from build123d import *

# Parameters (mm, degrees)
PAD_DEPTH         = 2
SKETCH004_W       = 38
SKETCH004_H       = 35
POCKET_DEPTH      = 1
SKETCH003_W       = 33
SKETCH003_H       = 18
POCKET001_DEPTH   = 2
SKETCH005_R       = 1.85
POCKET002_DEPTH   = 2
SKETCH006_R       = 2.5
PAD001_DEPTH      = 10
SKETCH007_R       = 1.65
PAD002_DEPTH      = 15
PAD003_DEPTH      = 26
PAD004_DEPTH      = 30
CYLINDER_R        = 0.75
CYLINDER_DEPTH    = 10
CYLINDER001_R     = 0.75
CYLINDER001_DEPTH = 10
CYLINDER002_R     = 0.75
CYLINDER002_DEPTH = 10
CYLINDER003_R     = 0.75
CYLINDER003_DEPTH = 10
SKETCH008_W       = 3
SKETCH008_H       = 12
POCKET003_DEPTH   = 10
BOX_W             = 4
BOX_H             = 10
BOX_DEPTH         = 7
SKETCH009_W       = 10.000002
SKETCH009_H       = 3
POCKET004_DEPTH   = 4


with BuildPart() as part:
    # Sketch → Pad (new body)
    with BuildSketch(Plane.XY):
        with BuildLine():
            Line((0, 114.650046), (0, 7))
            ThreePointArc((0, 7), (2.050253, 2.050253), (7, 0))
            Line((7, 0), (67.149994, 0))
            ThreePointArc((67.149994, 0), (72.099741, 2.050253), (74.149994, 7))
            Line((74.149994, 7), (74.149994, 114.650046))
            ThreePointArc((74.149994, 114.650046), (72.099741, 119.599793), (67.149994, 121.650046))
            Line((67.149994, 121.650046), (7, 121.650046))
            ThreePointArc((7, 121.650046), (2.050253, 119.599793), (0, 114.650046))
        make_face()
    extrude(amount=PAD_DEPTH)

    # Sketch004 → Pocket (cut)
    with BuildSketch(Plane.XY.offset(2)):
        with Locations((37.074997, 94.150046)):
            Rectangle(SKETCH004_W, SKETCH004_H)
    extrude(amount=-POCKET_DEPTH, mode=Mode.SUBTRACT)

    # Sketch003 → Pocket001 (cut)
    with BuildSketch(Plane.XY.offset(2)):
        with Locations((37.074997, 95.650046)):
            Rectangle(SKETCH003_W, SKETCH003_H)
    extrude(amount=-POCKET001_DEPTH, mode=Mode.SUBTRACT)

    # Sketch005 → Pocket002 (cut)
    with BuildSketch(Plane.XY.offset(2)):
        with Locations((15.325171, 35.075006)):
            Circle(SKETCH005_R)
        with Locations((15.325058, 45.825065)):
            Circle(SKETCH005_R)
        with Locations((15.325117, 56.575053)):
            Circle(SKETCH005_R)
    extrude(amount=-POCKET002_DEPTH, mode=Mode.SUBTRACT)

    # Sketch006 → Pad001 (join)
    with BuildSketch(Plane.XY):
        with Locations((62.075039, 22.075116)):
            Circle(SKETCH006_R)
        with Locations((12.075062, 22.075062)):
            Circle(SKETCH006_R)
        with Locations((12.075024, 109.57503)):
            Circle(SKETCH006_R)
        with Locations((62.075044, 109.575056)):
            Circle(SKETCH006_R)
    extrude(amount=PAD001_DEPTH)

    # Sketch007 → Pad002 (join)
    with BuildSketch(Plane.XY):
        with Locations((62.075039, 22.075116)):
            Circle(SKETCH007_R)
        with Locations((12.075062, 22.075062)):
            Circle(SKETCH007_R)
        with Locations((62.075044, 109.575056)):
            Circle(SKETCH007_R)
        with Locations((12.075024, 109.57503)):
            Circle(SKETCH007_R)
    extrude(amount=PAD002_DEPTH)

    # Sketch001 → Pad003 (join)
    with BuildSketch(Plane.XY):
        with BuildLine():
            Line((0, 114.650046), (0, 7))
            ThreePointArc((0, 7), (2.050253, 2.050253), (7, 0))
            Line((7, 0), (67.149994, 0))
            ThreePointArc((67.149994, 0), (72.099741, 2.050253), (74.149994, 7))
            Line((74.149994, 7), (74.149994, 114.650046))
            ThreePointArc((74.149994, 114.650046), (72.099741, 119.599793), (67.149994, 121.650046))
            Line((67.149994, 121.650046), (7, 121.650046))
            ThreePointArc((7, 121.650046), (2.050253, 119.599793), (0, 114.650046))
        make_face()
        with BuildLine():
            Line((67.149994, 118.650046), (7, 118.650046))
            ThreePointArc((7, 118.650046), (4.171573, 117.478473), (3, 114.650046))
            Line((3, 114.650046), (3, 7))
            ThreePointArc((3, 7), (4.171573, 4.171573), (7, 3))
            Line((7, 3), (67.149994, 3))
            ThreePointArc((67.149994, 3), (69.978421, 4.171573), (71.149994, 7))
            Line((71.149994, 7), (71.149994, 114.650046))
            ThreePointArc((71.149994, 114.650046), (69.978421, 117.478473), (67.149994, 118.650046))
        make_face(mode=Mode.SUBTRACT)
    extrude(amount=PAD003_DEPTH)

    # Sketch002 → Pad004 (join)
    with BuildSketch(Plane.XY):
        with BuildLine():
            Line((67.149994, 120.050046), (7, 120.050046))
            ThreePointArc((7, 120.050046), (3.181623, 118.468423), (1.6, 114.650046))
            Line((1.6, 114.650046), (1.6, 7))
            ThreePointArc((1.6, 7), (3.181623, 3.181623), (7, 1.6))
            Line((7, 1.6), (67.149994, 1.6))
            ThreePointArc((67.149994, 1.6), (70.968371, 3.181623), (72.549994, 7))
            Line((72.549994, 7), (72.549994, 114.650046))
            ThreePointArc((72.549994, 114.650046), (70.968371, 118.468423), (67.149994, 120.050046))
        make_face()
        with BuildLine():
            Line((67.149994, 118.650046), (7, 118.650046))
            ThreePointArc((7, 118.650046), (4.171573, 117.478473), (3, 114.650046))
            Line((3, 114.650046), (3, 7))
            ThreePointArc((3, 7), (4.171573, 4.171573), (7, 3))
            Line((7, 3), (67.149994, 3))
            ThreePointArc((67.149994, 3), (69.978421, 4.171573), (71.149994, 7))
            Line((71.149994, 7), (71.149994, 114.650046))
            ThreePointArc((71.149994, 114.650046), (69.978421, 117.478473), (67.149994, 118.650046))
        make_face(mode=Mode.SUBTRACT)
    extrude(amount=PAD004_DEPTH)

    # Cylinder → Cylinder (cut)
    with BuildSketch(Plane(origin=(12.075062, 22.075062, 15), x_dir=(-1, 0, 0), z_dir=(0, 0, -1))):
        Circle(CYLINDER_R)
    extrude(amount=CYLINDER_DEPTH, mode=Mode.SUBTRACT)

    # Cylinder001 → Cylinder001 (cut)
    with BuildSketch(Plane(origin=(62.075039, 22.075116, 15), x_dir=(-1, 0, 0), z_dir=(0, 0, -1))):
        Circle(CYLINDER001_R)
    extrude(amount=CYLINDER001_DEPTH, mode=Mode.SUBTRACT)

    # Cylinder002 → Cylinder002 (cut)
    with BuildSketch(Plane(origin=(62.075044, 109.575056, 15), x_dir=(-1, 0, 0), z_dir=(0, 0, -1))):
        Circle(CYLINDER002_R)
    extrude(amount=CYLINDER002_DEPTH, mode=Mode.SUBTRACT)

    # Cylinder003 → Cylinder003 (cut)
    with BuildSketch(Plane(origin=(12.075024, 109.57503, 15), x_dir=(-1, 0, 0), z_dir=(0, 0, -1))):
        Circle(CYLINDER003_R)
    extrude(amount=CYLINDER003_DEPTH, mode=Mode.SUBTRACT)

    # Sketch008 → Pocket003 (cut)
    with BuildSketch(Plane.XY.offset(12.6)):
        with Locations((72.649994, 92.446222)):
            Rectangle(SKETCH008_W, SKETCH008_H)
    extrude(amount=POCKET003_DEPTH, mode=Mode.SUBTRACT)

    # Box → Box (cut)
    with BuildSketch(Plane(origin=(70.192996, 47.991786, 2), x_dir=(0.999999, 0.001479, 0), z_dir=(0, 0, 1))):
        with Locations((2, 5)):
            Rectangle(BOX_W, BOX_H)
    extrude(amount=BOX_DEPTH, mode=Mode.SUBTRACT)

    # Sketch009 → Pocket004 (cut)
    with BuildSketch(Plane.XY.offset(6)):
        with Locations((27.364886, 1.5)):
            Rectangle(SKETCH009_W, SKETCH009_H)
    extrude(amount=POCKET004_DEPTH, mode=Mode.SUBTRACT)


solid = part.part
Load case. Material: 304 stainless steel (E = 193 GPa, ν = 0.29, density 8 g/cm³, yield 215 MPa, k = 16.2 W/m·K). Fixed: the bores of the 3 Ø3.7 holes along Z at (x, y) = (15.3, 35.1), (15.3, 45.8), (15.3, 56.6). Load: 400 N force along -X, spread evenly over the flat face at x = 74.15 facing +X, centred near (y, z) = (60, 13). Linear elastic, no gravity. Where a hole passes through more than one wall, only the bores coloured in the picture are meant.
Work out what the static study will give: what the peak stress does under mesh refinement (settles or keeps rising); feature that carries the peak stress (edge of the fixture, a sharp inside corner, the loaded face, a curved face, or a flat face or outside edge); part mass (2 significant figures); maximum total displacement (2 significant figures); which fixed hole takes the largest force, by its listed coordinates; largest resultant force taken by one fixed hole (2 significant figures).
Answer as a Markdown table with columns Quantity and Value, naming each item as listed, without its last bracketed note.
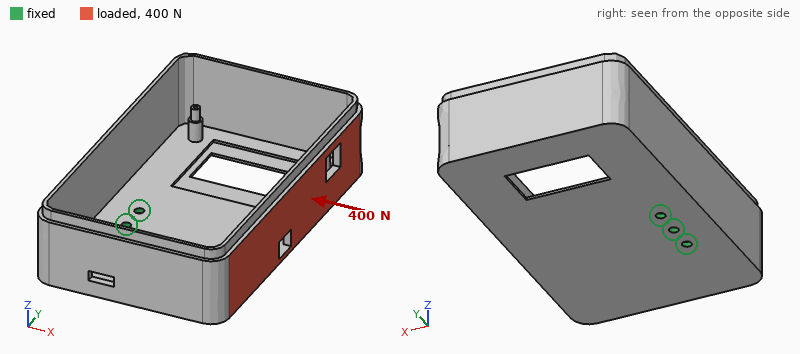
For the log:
| Quantity | Value |
|---|---|
| what the peak stress does under mesh refinement | keeps rising |
| feature that carries the peak stress | edge of the fixture |
| part mass | 360 g |
| maximum total displacement | 0.35 mm |
| which fixed hole takes the largest force, by its listed coordinates | (15.3, 56.6) |
| largest resultant force taken by one fixed hole | 390 N |
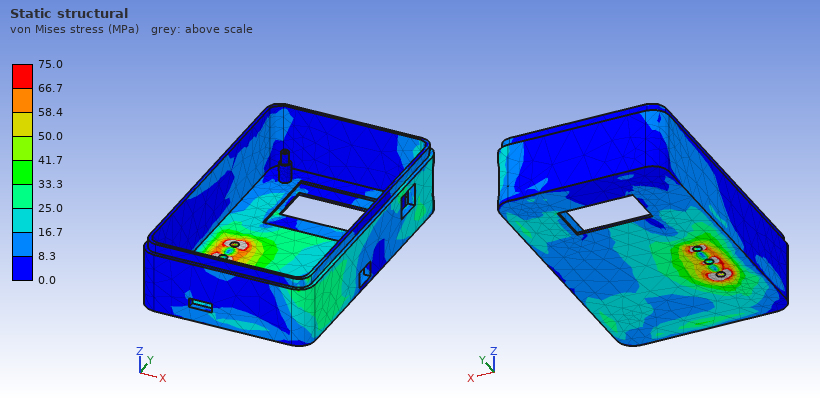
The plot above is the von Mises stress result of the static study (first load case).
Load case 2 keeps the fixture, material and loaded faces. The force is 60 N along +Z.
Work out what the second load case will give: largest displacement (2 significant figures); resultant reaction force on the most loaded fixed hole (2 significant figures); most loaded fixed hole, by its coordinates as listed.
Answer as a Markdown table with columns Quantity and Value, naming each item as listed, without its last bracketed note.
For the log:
| Quantity | Value |
|---|---|
| largest displacement | 0.26 mm |
| resultant reaction force on the most loaded fixed hole | 77 N |
| most loaded fixed hole, by its coordinates as listed | (15.3, 56.6) |
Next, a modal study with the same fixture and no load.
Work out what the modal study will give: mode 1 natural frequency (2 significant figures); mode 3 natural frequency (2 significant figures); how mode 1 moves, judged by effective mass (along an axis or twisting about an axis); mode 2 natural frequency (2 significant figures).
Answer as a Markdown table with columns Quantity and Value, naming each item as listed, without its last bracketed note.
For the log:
| Quantity | Value |
|---|---|
| mode 1 natural frequency | 220 Hz |
| mode 3 natural frequency | 730 Hz |
| how mode 1 moves, judged by effective mass | along Z |
| mode 2 natural frequency | 390 Hz |
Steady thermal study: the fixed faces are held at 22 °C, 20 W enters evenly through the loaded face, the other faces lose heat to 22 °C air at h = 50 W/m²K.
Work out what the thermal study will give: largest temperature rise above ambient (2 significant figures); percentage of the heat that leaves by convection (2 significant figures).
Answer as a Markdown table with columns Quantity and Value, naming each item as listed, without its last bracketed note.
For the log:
| Quantity | Value |
|---|---|
| largest temperature rise above ambient | 58 K |
| percentage of the heat that leaves by convection | 99 % |
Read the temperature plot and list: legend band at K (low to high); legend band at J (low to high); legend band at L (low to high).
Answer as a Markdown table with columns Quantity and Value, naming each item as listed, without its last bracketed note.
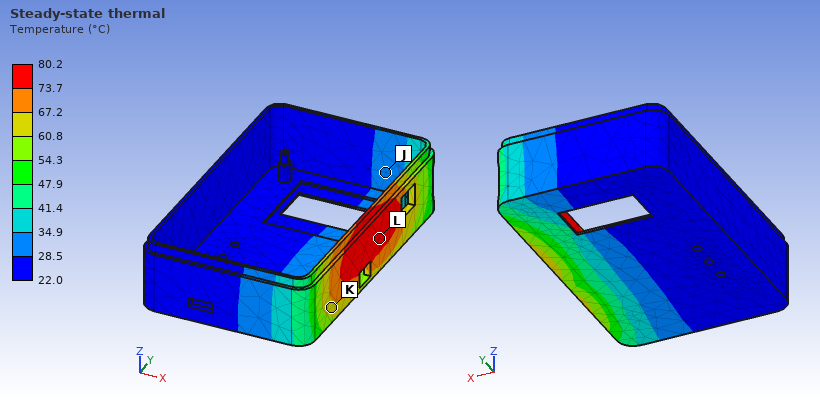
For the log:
| Quantity | Value |
|---|---|
| legend band at K | 60.8 to 67.2 °C |
| legend band at J | 28.5 to 34.9 °C |
| legend band at L | 73.7 to 80.2 °C |
